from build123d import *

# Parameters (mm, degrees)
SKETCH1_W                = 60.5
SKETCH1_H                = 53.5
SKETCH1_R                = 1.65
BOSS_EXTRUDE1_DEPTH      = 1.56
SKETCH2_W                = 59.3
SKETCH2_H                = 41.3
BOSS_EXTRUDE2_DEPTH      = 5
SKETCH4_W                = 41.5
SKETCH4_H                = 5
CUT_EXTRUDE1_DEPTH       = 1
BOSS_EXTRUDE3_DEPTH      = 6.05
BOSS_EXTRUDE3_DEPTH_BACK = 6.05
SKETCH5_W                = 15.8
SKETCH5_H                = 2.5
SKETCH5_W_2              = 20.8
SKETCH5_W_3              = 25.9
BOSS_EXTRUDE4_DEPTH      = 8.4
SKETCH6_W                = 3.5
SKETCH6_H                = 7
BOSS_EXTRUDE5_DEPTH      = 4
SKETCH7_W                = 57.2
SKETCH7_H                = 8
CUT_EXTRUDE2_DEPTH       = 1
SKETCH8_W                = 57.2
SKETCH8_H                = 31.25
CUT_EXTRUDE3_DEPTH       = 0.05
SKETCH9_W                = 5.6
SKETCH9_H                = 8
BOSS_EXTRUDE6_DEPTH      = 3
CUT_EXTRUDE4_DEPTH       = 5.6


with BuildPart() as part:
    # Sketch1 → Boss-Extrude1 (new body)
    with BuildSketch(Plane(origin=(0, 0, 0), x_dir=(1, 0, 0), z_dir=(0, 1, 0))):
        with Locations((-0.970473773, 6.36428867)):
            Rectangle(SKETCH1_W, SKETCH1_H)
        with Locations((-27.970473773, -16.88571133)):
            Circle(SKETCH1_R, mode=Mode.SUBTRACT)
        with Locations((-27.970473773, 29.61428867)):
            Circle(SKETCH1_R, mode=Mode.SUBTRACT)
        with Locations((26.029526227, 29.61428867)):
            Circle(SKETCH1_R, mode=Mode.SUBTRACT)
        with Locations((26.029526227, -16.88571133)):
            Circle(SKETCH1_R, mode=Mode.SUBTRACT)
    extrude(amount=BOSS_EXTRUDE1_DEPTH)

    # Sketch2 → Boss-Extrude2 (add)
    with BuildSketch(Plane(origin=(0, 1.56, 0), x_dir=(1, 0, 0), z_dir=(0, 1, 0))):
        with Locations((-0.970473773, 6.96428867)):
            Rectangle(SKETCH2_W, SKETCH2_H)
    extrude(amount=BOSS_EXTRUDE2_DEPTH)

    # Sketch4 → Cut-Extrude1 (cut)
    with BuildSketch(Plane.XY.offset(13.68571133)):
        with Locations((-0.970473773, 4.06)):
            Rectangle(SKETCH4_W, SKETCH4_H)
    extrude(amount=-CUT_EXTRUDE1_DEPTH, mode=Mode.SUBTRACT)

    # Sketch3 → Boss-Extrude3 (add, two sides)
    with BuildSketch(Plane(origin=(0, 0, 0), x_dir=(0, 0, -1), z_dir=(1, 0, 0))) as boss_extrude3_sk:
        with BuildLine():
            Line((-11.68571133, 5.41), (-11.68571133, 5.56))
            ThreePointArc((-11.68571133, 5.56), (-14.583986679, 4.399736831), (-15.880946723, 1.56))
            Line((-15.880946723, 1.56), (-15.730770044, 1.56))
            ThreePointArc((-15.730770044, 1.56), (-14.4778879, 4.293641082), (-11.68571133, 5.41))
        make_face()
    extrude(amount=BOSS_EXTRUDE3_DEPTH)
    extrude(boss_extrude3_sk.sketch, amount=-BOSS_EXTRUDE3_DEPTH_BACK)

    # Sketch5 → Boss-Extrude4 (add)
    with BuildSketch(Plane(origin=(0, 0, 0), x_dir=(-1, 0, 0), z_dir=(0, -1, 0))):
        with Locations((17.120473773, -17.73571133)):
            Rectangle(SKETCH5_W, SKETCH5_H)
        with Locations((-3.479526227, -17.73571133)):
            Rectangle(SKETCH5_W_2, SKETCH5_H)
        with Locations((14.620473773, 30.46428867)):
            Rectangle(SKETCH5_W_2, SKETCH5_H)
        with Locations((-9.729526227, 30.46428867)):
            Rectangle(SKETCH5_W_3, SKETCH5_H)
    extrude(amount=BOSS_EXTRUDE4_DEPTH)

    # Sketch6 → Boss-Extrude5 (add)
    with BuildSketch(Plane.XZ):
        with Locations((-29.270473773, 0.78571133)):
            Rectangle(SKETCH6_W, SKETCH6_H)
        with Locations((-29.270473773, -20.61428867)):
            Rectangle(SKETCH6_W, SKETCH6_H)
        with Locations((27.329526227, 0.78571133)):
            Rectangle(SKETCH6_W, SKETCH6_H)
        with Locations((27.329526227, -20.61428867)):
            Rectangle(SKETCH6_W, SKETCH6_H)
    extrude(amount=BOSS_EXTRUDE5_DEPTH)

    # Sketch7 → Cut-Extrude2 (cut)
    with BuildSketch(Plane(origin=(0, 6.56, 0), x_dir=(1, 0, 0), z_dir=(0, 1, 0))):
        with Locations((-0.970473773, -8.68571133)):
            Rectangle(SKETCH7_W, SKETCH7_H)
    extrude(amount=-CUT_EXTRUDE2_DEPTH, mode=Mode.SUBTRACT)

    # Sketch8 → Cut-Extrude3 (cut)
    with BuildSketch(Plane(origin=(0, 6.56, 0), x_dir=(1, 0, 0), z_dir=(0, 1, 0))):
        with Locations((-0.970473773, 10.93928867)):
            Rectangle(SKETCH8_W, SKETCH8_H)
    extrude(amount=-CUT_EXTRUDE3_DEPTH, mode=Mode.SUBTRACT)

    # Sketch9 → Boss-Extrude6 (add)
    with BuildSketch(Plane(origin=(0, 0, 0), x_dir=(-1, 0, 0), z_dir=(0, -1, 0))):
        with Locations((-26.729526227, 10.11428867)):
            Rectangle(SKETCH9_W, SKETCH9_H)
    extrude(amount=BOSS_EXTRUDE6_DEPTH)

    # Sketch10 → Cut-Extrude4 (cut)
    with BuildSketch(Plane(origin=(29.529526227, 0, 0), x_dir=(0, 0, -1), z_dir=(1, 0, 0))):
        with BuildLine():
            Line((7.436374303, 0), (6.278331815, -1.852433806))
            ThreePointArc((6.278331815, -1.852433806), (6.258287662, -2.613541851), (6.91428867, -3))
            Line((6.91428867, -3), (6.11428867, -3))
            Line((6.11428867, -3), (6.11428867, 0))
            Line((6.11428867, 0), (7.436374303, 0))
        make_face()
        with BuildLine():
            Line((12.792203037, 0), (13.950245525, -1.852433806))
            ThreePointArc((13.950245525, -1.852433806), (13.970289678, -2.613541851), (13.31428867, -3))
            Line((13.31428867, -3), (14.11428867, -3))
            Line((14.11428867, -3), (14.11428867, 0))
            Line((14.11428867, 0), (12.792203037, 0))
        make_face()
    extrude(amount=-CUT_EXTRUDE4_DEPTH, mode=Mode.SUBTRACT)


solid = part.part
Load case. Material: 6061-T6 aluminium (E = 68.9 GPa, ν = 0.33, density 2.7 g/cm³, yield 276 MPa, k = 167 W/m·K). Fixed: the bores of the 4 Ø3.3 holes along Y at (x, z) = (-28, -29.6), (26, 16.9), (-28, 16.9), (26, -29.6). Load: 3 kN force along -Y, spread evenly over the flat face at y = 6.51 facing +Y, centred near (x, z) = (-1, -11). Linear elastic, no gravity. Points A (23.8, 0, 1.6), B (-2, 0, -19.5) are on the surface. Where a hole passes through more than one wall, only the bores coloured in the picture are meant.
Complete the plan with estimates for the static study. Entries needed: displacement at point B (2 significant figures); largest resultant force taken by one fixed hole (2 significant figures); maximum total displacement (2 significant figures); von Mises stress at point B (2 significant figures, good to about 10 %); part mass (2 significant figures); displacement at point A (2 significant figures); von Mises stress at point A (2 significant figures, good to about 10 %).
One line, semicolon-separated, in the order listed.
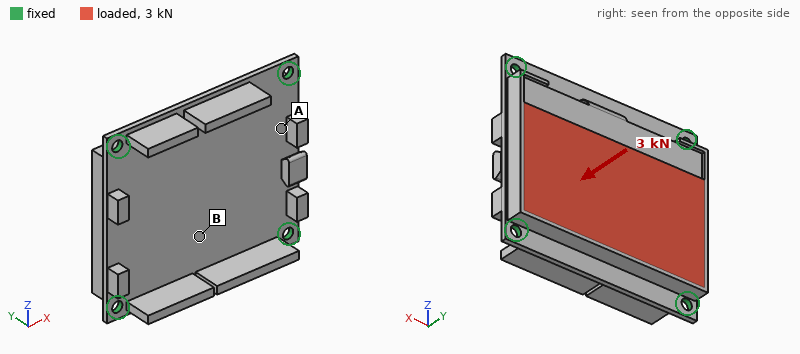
77 µm; 1.5 kN; 87 µm; 38 MPa; 51 g; 42 µm; 20 MPa
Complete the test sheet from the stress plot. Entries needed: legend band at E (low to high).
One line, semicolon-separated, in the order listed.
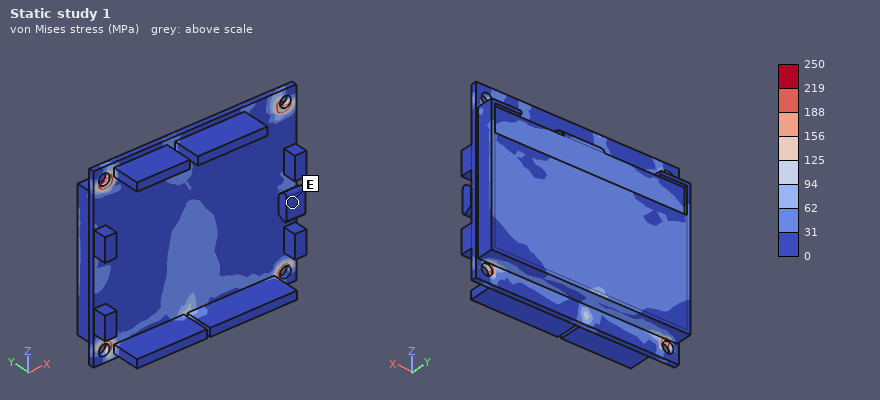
0 to 31 MPa
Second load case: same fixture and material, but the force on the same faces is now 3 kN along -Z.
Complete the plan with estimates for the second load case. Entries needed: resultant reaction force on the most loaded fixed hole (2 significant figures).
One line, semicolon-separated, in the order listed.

830 N
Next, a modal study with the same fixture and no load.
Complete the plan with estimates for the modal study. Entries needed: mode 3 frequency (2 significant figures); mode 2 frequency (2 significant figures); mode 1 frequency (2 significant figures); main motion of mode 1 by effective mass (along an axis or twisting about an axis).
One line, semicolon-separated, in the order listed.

8300 Hz; 6700 Hz; 4800 Hz; along Y
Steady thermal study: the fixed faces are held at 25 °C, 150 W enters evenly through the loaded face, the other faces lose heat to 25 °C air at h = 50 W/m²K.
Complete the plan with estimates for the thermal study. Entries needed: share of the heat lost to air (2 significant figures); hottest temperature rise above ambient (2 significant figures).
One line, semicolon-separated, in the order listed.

13 %; 67 K
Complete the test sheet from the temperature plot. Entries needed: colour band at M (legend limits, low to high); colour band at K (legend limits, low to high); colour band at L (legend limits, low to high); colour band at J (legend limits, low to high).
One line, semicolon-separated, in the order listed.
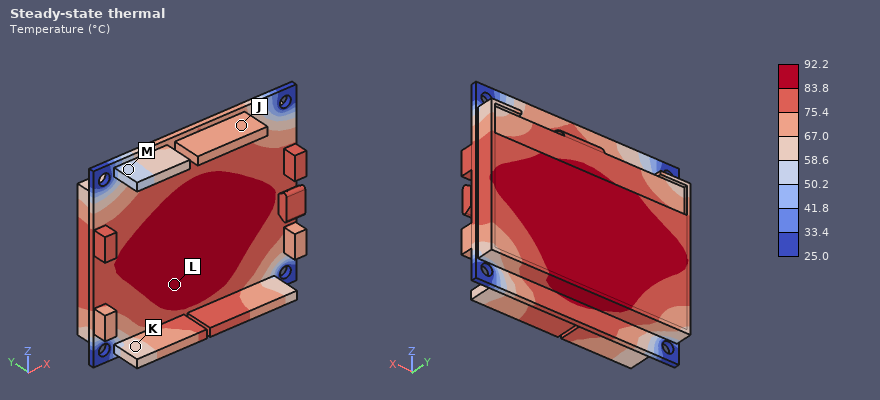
50.2 to 58.6 °C; 58.6 to 67.0 °C; 83.8 to 92.2 °C; 67.0 to 75.4 °C
